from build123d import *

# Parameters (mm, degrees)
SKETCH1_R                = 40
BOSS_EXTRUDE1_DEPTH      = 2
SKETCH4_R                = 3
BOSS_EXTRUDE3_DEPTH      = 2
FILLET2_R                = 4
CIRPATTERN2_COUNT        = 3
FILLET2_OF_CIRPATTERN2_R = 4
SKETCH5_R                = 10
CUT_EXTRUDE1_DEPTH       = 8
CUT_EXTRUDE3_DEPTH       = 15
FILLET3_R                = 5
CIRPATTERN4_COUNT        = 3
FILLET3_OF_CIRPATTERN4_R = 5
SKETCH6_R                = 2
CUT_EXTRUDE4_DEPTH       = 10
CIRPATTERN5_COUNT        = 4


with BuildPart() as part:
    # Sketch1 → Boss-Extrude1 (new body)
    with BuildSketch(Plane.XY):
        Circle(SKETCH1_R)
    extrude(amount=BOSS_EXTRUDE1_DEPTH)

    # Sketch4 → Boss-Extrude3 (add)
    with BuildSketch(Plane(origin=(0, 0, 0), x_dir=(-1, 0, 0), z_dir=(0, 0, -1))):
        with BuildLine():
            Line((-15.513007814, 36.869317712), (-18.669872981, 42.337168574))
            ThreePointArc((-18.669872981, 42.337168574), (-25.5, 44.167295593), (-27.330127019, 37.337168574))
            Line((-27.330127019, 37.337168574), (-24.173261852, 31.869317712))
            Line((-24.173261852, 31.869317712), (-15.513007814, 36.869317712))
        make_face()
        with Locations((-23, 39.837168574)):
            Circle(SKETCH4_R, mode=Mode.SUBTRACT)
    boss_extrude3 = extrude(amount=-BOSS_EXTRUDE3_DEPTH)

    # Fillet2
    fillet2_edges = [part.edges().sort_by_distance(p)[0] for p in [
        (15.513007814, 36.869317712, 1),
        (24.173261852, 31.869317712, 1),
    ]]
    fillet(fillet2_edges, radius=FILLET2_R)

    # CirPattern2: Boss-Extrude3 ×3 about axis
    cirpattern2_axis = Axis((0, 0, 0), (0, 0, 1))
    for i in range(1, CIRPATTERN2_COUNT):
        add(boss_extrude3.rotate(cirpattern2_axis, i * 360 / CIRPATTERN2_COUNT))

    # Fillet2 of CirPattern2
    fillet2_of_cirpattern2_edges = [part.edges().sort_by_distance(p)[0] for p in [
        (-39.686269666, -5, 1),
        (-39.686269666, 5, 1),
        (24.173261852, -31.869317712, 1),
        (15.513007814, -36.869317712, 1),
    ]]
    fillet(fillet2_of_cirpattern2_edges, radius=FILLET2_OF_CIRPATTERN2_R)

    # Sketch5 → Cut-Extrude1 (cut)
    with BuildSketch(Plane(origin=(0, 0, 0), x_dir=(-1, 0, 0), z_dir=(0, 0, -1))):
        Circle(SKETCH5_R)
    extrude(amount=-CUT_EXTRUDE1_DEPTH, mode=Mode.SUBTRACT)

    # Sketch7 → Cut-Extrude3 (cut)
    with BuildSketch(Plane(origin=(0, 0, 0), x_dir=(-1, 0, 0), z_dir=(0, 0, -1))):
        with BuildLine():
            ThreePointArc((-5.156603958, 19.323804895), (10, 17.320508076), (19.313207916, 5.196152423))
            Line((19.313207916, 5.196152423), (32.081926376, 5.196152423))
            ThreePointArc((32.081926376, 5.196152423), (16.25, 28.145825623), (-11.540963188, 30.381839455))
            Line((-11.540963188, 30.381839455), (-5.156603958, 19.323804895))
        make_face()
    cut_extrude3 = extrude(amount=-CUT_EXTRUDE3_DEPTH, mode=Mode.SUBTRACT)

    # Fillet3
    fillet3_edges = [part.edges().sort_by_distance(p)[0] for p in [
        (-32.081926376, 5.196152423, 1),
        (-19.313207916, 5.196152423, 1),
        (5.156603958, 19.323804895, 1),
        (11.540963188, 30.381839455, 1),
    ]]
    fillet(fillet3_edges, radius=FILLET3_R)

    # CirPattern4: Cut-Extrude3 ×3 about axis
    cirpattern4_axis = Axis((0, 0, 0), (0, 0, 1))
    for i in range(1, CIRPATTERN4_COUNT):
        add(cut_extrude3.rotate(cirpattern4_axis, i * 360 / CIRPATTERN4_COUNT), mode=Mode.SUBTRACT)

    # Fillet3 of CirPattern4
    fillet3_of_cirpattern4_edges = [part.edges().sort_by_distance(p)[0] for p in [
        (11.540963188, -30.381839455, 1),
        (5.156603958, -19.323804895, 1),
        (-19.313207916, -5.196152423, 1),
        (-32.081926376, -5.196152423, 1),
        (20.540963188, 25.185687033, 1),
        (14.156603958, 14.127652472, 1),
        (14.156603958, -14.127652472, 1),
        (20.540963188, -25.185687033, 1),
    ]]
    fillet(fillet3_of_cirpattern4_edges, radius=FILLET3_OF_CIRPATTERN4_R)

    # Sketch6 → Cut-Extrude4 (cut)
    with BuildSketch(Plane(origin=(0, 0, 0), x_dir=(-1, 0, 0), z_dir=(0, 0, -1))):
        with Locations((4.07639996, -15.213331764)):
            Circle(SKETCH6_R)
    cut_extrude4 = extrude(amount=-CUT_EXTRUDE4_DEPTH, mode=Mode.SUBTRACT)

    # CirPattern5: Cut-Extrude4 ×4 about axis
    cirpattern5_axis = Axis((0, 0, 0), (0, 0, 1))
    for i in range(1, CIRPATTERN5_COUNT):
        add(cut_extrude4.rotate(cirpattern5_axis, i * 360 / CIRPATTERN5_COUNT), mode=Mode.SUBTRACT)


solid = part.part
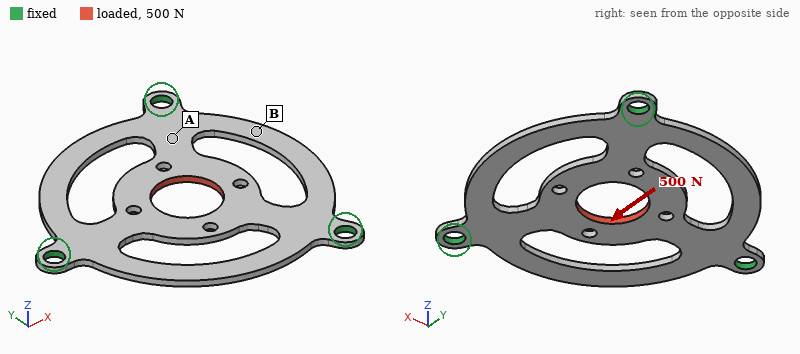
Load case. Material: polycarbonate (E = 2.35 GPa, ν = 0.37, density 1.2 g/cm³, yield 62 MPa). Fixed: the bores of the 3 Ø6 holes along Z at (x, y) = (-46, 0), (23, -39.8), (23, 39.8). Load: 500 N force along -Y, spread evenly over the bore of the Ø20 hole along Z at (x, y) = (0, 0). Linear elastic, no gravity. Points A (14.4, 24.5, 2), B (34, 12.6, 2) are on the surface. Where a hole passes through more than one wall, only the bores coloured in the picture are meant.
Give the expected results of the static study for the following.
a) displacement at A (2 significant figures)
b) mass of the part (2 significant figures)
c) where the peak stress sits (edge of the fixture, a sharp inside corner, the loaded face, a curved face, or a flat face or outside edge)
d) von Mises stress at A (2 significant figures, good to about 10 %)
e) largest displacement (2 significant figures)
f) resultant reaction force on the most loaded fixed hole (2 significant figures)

0.11 mm
7.9 g
a curved face
9.4 MPa
0.45 mm
230 N
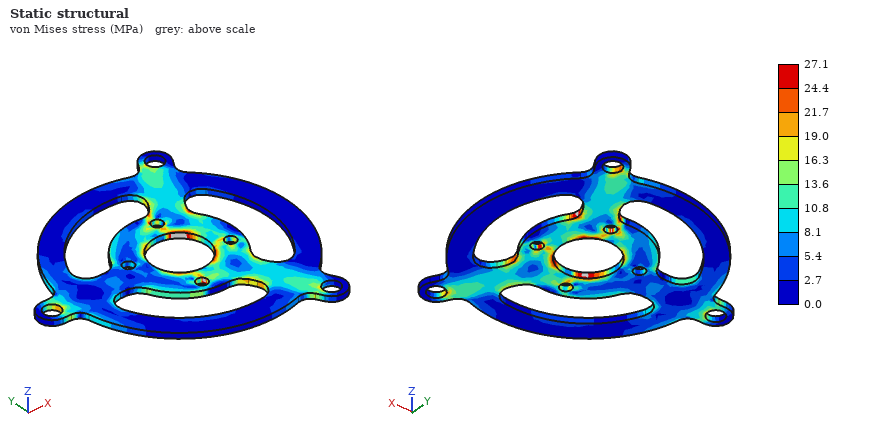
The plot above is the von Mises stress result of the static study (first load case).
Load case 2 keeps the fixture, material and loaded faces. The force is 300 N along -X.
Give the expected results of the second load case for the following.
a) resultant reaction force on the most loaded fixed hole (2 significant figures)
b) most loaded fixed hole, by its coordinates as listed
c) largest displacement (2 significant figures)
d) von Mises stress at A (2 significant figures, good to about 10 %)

160 N
(-46, 0)
0.28 mm
3.7 MPa
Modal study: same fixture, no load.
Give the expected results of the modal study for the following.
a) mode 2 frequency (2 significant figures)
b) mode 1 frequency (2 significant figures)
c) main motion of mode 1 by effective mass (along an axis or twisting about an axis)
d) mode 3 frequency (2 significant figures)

430 Hz
410 Hz
along Z
430 Hz
